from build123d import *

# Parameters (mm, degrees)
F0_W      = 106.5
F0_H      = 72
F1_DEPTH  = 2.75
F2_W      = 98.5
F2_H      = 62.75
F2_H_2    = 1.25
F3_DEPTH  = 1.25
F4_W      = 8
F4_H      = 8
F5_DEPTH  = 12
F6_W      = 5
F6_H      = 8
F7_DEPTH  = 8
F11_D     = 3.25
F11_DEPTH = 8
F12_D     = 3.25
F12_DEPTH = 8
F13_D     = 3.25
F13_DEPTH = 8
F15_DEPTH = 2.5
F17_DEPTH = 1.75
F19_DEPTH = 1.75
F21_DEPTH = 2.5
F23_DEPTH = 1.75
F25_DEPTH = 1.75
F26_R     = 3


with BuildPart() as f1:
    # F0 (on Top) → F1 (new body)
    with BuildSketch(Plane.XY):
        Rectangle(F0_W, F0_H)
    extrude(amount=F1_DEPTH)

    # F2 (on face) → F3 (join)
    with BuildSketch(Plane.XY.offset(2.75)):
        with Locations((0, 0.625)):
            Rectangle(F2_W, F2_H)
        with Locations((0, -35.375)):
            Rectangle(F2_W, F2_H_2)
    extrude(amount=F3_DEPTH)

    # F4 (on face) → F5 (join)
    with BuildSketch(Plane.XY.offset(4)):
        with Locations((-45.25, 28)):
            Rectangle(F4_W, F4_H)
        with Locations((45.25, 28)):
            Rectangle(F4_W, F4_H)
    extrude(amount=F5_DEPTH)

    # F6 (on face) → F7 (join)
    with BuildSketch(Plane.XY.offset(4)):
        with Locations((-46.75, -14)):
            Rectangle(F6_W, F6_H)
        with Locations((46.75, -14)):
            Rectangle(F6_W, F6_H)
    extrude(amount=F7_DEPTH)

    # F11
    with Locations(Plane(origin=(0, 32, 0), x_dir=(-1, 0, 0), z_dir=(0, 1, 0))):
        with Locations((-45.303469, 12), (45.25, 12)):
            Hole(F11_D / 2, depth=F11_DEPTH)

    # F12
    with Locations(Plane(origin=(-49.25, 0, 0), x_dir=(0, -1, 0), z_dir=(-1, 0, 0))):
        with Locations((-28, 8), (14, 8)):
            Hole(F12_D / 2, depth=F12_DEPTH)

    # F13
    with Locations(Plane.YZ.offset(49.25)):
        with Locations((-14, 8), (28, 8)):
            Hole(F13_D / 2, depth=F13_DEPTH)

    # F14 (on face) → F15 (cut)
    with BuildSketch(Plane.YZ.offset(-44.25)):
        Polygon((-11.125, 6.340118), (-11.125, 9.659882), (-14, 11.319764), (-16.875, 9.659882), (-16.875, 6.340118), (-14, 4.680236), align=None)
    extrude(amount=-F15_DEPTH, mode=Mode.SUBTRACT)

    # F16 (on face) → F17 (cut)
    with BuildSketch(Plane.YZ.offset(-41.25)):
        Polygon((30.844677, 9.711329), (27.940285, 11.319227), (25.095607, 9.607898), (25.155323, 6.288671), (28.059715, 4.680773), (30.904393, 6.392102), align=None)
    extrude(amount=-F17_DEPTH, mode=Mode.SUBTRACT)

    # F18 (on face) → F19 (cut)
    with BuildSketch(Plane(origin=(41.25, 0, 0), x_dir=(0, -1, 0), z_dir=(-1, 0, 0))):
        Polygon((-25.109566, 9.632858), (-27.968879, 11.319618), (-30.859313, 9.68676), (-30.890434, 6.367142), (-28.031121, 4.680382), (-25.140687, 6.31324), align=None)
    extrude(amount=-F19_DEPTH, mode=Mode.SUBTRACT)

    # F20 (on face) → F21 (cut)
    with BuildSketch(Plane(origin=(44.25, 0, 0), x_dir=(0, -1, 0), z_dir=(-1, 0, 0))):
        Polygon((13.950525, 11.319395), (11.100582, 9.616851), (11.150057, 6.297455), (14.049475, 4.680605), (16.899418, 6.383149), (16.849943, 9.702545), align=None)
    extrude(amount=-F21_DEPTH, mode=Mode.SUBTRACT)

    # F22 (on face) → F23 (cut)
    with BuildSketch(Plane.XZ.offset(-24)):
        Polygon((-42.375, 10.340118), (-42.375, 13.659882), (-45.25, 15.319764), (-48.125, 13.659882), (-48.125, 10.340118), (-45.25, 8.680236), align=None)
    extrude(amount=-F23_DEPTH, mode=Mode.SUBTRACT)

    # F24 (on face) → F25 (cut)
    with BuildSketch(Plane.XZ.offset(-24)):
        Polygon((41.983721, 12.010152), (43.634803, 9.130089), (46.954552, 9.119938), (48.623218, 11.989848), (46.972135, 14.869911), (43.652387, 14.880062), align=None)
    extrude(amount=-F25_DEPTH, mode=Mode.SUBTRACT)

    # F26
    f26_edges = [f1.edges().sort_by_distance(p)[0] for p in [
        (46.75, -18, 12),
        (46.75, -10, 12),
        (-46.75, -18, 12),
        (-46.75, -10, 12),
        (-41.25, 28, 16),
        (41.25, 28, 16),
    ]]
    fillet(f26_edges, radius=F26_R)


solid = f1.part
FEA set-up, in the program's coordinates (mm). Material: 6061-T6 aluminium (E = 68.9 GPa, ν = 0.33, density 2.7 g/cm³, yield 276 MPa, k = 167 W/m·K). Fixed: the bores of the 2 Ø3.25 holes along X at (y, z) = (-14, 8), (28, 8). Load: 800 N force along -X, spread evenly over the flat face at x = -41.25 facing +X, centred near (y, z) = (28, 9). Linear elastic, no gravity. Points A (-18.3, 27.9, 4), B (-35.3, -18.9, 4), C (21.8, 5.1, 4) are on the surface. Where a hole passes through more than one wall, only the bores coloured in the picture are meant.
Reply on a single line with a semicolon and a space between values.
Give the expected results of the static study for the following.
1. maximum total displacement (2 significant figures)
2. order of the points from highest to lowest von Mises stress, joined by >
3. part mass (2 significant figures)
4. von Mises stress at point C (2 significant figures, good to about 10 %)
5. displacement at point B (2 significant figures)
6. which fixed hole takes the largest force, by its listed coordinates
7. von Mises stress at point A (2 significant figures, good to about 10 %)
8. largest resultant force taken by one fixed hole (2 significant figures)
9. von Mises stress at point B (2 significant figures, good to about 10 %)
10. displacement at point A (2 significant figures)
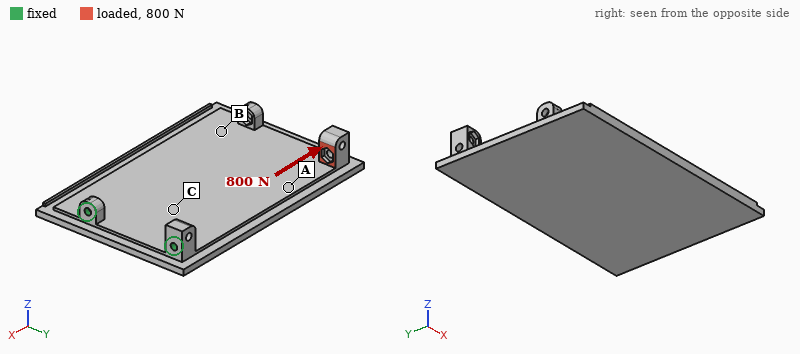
1.4 mm; A > C > B; 82 g; 32 MPa; 0.93 mm; (28, 8); 53 MPa; 780 N; 16 MPa; 0.59 mm
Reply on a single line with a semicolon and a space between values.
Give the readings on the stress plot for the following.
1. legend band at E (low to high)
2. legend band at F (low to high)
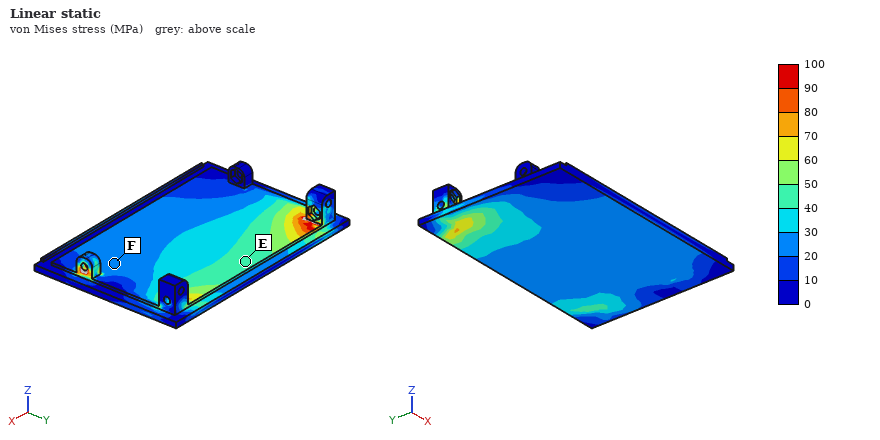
40 to 50 MPa; 20 to 30 MPa
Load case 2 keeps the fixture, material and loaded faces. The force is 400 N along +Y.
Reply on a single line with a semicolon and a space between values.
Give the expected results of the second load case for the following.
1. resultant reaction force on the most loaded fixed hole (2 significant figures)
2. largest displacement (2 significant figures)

840 N; 0.53 mm
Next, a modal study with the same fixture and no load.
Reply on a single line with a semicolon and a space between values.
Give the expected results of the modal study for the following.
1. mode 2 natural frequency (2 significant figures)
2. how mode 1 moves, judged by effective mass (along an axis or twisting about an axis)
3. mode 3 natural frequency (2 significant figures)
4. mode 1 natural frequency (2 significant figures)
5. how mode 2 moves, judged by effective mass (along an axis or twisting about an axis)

900 Hz; along Z; 1700 Hz; 250 Hz; twisting about X
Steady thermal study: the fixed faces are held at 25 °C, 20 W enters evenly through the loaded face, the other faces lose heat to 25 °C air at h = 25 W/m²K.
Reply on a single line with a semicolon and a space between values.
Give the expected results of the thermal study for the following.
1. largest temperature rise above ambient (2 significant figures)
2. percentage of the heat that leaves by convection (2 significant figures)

73 K; 43 %
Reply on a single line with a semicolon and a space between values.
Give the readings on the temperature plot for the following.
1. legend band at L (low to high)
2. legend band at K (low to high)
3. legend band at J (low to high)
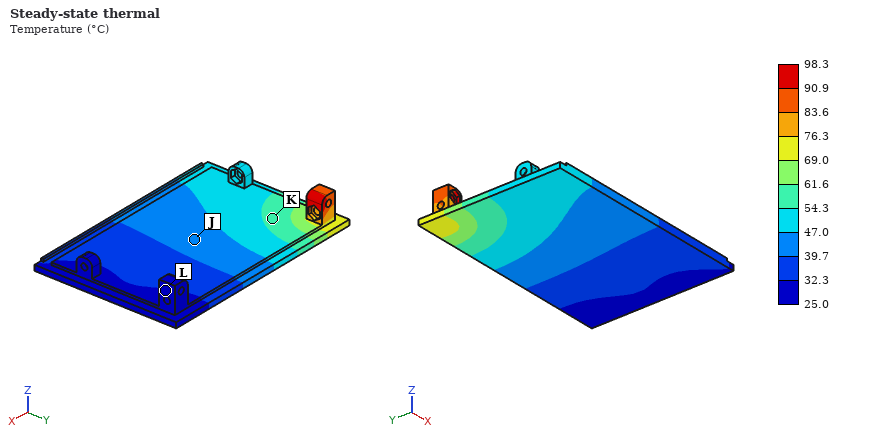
25.0 to 32.3 °C; 54.3 to 61.6 °C; 39.7 to 47.0 °C
